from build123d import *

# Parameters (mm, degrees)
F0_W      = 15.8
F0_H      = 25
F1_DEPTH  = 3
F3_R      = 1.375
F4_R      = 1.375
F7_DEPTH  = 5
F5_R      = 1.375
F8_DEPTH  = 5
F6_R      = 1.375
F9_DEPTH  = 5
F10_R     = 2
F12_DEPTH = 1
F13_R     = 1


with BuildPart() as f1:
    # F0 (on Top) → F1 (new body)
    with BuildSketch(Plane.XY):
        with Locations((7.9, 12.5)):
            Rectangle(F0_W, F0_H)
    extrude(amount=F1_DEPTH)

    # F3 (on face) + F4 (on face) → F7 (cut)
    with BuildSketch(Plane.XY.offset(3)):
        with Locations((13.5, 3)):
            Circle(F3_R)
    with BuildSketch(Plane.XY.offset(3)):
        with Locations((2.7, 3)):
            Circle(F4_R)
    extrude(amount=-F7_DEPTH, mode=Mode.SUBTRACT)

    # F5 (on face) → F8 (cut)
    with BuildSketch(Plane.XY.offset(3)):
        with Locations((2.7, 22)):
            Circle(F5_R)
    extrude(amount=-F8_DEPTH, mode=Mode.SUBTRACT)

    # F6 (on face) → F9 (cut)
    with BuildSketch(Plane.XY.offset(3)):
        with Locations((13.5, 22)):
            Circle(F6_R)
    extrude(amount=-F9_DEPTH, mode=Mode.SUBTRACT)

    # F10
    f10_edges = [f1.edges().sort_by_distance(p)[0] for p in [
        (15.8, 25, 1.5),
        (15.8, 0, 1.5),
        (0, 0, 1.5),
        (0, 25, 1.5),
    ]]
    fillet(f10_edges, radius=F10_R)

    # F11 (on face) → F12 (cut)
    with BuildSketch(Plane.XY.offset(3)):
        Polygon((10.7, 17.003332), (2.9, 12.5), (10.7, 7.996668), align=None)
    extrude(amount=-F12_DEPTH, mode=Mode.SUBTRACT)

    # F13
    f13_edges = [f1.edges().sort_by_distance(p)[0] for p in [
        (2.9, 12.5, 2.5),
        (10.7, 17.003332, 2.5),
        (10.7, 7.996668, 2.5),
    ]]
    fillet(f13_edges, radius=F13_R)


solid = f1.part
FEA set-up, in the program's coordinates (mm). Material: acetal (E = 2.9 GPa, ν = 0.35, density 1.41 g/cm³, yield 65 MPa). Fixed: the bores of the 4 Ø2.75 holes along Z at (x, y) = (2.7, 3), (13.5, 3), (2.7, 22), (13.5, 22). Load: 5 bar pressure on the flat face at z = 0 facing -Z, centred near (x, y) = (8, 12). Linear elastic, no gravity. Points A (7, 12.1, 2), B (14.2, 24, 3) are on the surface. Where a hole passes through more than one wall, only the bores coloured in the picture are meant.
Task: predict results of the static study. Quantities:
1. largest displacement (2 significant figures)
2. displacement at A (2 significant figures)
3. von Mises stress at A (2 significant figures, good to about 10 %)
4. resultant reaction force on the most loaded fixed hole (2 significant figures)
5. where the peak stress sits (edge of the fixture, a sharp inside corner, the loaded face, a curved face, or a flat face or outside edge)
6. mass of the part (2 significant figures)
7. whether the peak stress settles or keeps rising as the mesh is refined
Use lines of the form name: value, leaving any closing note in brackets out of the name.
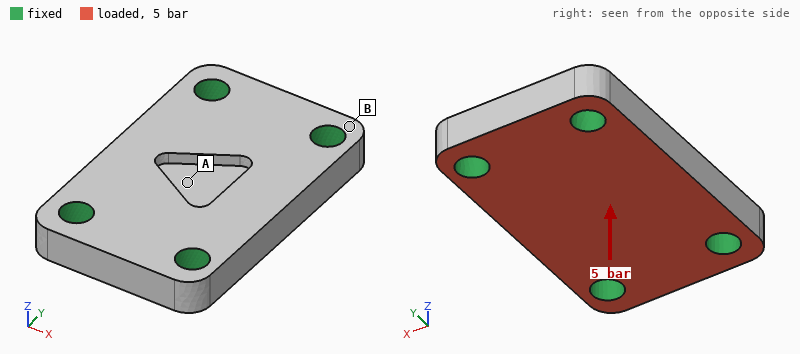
largest displacement: 34 µm
displacement at A: 34 µm
von Mises stress at A: 3.4 MPa
resultant reaction force on the most loaded fixed hole: 48 N
where the peak stress sits: edge of the fixture
mass of the part: 1.5 g
whether the peak stress settles or keeps rising as the mesh is refined: keeps rising
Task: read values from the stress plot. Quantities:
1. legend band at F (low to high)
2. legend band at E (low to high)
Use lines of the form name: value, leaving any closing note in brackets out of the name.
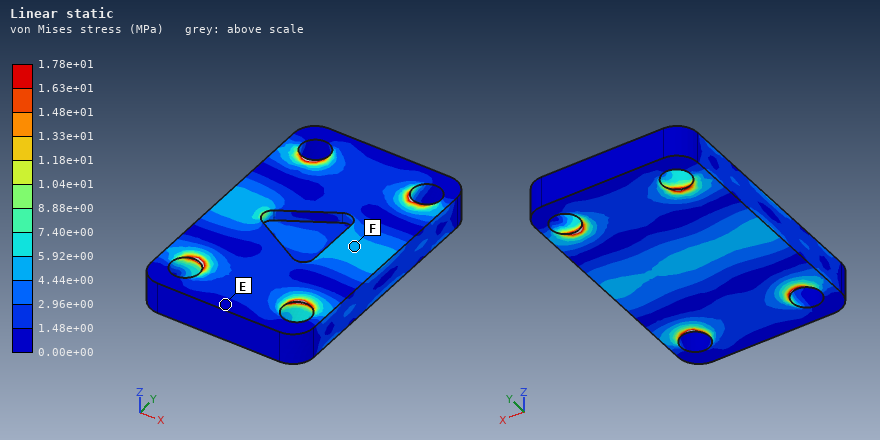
legend band at F: 4.44e+00 to 5.92e+00 MPa
legend band at E: 0.00e+00 to 1.48e+00 MPa
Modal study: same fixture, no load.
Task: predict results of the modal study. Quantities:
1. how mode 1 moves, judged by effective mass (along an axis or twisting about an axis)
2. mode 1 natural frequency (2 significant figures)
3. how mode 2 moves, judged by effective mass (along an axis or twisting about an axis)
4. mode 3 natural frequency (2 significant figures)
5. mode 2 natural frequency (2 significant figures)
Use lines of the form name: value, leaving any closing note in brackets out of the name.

how mode 1 moves, judged by effective mass: along Z
mode 1 natural frequency: 11 kHz
how mode 2 moves, judged by effective mass: twisting about Y
mode 3 natural frequency: 22 kHz
mode 2 natural frequency: 15 kHz
